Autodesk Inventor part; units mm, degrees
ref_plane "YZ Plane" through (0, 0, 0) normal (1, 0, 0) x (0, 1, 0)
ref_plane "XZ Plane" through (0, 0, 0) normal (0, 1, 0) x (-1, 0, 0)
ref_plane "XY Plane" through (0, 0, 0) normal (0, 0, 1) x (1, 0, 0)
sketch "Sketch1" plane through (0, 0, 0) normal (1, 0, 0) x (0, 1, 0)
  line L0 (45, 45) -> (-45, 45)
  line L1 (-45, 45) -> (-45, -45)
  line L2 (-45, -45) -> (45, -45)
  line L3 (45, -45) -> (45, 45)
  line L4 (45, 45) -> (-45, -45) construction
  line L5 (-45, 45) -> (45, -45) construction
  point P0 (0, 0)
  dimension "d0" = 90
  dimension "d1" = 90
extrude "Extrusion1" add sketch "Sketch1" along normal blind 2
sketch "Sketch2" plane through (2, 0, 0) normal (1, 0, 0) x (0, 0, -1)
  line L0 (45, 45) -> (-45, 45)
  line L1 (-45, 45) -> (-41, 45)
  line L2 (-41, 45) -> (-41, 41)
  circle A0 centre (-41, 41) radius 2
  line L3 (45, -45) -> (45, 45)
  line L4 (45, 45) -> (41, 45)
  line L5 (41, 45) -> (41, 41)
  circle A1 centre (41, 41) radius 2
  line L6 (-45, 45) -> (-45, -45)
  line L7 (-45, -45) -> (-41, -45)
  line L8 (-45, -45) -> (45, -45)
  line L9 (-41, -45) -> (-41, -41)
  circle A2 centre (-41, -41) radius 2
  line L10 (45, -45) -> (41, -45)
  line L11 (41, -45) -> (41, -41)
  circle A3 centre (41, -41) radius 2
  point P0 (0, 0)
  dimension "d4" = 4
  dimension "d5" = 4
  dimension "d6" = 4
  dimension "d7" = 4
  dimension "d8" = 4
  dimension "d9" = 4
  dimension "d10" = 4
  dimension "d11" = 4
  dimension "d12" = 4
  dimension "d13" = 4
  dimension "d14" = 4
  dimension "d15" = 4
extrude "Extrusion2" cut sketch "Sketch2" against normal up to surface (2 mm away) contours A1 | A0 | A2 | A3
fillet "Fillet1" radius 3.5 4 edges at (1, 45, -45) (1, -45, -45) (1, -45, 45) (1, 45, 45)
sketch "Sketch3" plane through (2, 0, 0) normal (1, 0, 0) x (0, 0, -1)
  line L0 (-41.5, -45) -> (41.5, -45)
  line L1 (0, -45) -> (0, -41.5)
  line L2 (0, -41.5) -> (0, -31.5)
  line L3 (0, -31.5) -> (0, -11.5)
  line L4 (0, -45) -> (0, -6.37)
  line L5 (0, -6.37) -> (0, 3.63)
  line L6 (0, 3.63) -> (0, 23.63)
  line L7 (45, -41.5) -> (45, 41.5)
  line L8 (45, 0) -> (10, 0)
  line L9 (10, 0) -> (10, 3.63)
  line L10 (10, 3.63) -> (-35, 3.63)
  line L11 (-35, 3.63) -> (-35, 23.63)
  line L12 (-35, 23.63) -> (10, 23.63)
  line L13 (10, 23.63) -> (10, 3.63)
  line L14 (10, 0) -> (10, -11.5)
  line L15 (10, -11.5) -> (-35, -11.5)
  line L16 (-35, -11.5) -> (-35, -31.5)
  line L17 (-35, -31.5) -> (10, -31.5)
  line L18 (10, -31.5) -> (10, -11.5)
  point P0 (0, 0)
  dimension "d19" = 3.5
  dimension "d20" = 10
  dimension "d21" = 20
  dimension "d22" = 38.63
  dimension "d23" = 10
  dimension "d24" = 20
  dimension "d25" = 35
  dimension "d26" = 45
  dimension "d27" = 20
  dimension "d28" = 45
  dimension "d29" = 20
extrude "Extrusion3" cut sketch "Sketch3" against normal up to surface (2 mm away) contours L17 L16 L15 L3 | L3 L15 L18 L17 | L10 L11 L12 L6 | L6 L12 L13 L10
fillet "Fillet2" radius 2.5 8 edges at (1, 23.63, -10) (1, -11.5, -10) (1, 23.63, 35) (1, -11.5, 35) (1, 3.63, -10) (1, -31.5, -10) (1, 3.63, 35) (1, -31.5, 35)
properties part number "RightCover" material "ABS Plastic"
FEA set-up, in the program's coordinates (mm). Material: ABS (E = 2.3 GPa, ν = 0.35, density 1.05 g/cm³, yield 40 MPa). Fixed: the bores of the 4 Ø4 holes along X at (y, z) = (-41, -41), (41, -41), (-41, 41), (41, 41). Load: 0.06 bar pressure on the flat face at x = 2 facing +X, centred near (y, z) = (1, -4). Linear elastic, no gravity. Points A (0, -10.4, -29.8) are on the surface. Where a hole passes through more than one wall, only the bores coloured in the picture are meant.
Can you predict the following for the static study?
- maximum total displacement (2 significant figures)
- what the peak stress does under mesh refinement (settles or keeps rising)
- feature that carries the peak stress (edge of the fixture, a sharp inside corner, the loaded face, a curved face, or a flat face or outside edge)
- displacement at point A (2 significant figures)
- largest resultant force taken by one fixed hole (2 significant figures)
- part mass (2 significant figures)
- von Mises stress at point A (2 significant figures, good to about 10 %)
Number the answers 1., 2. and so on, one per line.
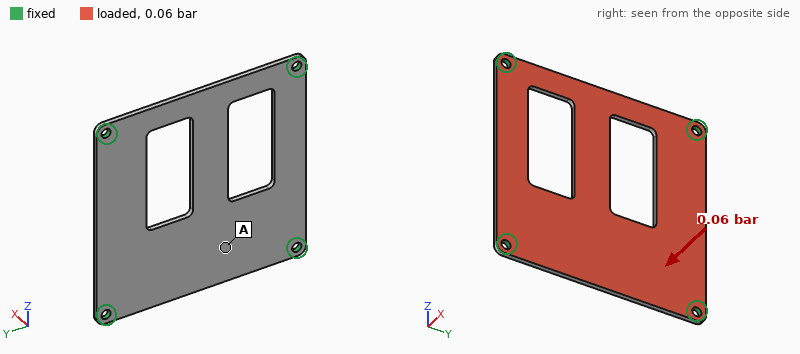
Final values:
1. 1.5 mm
2. keeps rising
3. edge of the fixture
4. 0.81 mm
5. 11 N
6. 13 g
7. 2.7 MPa
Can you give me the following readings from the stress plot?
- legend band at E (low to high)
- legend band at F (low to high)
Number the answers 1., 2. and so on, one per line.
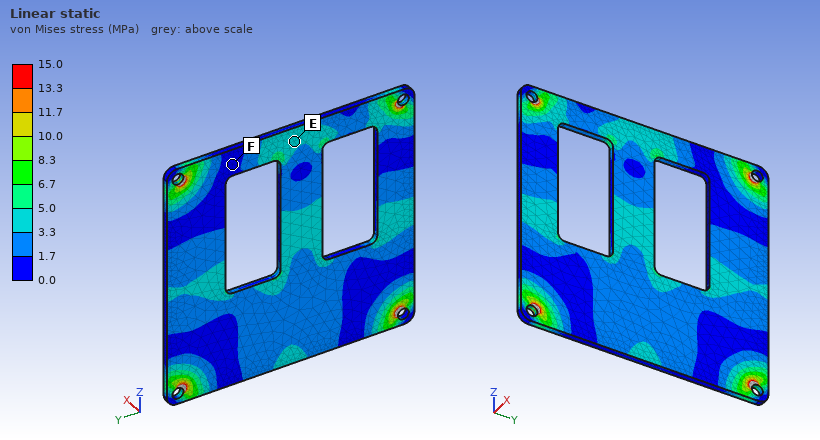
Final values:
1. 3.3 to 5.0 MPa
2. 0.0 to 1.7 MPa
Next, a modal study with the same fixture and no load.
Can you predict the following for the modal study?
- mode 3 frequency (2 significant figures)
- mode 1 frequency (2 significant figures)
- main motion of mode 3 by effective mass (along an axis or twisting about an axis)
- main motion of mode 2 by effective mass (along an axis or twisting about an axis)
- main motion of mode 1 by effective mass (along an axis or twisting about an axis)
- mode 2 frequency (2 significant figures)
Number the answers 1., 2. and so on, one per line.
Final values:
1. 500 Hz
2. 290 Hz
3. twisting about Z
4. twisting about Y
5. along X
6. 470 Hz
